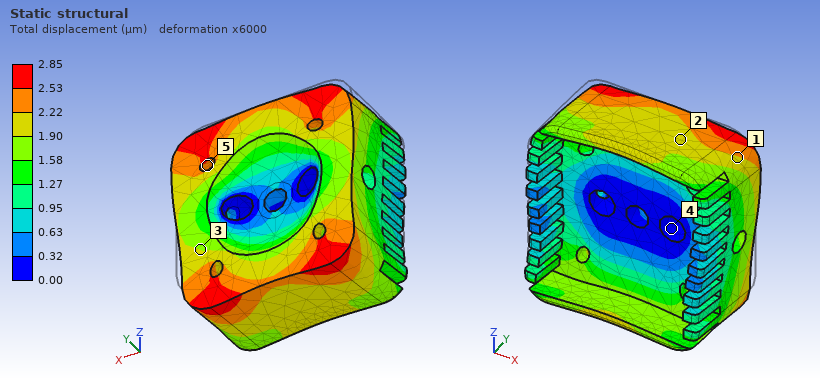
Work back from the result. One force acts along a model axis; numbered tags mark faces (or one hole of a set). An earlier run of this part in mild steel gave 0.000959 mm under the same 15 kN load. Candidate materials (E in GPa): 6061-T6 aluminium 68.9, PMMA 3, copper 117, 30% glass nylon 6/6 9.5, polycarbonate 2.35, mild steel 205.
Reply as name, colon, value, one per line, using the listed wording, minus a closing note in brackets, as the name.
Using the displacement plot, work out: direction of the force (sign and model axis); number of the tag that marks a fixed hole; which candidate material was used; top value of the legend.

direction of the force: -Z
number of the tag that marks a fixed hole: 4
which candidate material was used: 6061-T6 aluminium
top value of the legend: 2.85 µm
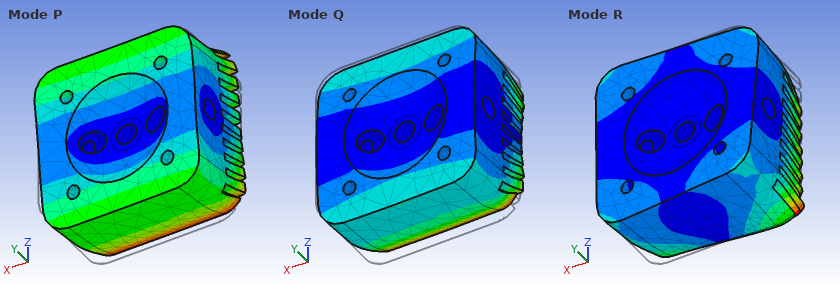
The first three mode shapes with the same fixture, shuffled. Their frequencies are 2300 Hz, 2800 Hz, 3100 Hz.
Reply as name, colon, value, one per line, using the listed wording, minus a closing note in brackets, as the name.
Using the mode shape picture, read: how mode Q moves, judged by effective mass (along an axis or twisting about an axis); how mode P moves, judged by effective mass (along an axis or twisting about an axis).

how mode Q moves, judged by effective mass: along Y
how mode P moves, judged by effective mass: twisting about X
